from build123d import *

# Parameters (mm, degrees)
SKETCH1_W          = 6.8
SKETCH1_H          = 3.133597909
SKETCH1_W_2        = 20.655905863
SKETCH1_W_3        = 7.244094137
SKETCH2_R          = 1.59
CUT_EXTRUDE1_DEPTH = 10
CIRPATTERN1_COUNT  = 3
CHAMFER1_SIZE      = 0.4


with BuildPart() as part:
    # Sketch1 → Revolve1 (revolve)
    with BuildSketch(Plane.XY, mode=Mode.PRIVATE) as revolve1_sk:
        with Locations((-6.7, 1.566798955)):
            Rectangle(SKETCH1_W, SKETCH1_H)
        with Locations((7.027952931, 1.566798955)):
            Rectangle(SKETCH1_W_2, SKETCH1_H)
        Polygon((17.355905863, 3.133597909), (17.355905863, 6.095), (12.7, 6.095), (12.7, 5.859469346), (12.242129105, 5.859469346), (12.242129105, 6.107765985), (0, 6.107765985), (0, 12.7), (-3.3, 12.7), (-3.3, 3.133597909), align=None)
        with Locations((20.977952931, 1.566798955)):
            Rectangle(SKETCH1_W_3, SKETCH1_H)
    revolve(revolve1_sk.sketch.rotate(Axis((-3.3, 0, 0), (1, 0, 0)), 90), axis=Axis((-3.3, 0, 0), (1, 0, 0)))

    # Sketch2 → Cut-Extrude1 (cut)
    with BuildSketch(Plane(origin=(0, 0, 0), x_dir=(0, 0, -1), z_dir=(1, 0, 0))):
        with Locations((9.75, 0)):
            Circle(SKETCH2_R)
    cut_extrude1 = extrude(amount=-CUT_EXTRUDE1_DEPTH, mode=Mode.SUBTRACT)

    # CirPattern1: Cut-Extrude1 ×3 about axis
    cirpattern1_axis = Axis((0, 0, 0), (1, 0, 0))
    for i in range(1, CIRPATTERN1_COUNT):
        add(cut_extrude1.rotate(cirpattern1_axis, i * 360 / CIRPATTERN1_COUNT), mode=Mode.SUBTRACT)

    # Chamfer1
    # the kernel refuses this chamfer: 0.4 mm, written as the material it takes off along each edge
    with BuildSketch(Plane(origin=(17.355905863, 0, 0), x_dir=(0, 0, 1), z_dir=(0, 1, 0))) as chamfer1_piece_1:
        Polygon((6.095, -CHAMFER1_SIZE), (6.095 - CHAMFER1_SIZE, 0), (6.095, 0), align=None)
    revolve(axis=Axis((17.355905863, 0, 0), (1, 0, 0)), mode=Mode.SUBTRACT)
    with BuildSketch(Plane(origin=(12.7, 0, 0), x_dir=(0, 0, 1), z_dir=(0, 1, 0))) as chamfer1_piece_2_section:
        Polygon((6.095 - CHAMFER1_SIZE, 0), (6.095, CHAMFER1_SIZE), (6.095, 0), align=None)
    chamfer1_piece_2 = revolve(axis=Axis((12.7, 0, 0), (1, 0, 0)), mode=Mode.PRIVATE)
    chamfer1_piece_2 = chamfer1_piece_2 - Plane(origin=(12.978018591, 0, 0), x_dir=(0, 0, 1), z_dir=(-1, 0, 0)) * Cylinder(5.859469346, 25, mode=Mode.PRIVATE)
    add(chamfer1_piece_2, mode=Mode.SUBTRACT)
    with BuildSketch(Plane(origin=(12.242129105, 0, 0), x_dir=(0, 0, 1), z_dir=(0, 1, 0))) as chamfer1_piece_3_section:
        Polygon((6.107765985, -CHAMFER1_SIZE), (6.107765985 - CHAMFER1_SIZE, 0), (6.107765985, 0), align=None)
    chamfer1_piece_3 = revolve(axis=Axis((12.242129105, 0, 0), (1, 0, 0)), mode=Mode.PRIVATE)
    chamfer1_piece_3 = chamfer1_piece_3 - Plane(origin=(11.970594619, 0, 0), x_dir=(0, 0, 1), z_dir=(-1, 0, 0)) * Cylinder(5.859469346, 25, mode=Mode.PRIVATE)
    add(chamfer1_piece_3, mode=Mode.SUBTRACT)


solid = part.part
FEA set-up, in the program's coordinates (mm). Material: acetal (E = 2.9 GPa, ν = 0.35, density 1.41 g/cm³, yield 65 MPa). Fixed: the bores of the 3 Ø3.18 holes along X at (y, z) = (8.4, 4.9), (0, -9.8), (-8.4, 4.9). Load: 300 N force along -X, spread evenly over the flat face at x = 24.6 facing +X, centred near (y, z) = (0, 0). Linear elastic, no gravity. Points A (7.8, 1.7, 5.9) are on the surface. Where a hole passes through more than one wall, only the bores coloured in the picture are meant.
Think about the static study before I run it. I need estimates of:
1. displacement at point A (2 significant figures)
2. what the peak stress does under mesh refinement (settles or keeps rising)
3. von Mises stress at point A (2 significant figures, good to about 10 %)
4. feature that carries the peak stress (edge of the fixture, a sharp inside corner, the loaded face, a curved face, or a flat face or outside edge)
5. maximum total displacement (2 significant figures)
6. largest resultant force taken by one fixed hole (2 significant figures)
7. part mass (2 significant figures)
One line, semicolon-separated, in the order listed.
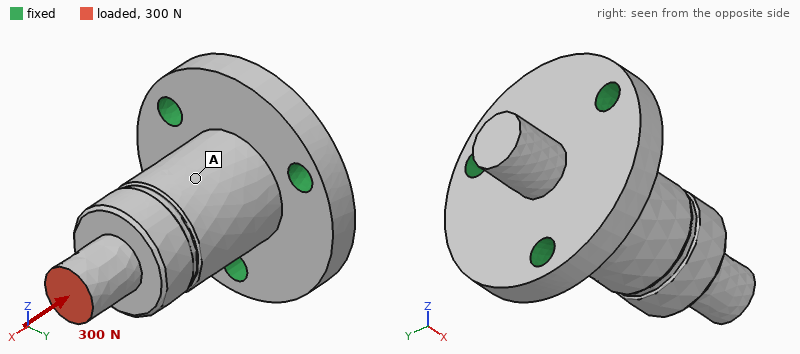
30 µm; keeps rising; 2.5 MPa; edge of the fixture; 67 µm; 100 N; 5.7 g
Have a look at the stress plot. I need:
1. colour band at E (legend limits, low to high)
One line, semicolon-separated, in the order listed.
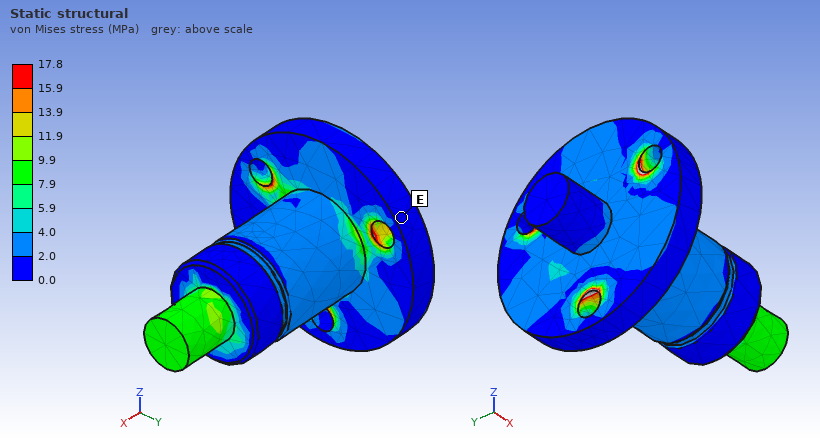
0.0 to 2.0 MPa
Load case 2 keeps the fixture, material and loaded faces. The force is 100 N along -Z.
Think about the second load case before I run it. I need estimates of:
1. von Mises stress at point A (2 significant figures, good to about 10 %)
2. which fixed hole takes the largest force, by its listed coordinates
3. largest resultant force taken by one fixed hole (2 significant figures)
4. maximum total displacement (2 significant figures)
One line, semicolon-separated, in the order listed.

8.9 MPa; (0, -9.8); 200 N; 0.45 mm
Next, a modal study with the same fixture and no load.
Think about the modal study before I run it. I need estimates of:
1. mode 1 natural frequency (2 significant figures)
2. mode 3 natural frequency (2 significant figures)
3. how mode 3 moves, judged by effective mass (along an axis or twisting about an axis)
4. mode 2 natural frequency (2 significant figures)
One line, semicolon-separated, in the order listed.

3300 Hz; 7900 Hz; along X; 3300 Hz
